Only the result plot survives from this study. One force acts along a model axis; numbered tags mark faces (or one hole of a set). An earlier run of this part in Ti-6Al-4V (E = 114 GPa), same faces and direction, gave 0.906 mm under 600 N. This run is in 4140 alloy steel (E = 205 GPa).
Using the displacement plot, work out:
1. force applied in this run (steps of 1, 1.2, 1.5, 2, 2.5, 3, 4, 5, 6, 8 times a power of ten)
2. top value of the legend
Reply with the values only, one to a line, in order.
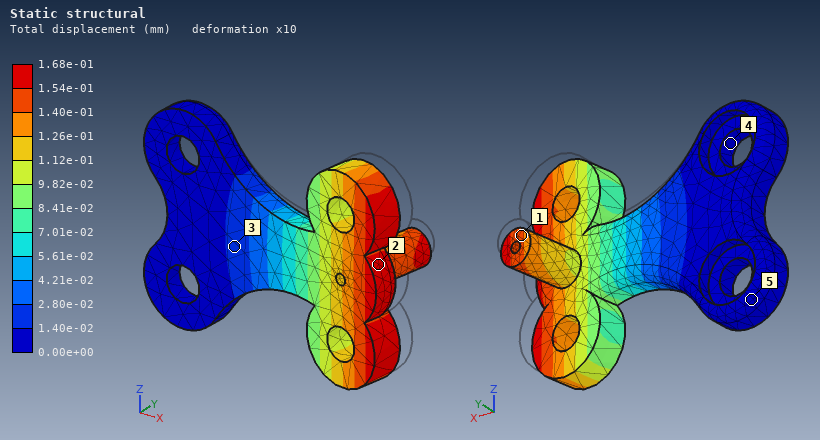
200 N
1.68e-01 mm
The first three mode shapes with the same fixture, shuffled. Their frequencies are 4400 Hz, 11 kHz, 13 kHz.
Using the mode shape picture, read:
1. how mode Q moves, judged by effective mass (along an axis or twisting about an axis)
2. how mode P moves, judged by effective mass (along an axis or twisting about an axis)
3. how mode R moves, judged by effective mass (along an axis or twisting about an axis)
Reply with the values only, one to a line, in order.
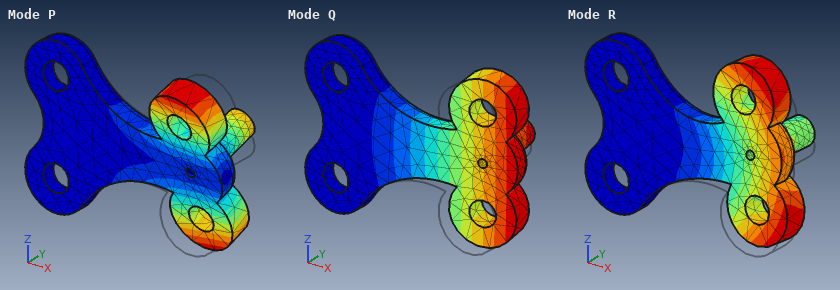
along Y
twisting about X
along Z
